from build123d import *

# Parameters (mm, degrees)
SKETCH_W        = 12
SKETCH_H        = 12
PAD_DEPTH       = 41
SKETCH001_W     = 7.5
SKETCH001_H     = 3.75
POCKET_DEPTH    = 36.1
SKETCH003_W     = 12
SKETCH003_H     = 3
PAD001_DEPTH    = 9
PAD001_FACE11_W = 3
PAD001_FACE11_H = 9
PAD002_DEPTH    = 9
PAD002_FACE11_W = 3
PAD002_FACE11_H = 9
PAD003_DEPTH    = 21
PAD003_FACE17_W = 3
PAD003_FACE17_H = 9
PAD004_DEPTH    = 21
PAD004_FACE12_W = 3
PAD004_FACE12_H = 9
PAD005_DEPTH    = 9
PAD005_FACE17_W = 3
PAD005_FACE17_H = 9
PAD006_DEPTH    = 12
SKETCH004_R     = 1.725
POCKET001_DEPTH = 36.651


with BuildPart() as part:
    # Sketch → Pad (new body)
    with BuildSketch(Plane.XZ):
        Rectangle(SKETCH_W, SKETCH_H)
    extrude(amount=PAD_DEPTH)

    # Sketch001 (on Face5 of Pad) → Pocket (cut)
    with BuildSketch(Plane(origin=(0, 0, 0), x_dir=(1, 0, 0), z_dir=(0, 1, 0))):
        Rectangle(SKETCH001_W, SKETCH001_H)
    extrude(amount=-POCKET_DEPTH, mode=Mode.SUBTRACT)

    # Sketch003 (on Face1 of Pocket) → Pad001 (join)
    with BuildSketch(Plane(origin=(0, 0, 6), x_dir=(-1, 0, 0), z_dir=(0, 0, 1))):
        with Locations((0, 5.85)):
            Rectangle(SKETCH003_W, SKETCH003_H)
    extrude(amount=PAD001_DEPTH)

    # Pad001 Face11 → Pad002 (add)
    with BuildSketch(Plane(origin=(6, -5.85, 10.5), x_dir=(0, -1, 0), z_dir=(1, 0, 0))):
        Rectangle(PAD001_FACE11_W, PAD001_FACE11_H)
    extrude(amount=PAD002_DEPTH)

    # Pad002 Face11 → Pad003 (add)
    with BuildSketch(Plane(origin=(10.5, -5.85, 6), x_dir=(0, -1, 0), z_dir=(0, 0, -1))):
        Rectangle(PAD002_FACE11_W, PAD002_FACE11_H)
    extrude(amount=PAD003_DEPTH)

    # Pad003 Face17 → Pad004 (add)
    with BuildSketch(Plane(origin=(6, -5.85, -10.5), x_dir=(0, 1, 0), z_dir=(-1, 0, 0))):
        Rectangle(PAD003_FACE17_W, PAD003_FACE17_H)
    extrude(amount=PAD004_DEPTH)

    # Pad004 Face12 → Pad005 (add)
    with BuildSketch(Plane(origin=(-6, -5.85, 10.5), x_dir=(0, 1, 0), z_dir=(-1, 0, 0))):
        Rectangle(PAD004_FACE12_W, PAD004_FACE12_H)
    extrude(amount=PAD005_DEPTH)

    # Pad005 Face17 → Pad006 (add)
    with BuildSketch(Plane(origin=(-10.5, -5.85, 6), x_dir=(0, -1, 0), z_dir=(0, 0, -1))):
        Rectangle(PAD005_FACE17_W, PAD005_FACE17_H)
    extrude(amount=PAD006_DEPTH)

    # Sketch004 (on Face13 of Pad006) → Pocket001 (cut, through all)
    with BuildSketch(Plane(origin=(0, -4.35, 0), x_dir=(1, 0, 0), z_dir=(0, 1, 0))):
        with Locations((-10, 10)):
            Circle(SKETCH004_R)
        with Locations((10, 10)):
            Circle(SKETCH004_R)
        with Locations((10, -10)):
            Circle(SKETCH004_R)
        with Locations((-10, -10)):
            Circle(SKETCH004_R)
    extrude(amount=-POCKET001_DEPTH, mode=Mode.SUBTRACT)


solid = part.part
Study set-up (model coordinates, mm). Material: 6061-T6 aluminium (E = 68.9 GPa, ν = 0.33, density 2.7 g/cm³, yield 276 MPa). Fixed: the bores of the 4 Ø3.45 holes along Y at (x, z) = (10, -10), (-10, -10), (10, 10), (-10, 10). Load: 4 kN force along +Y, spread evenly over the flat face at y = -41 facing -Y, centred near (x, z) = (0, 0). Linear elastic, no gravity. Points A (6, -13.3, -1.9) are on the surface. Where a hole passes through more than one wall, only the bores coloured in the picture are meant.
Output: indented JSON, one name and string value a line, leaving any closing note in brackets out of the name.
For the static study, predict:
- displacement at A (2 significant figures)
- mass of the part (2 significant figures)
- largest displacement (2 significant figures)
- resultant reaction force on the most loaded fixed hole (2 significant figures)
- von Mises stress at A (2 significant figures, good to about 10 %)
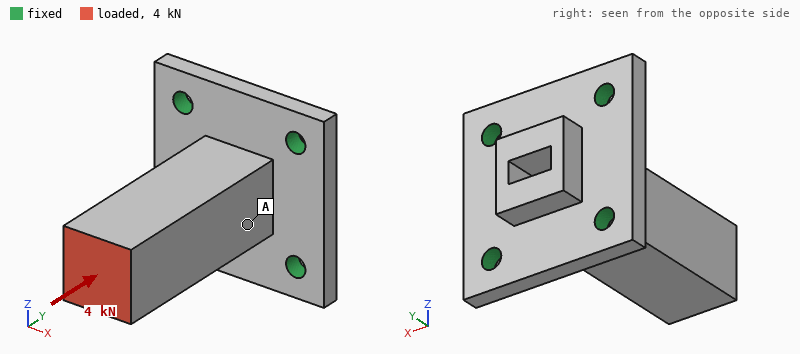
{
  "displacement at A": "30 µm",
  "mass of the part": "19 g",
  "largest displacement": "44 µm",
  "resultant reaction force on the most loaded fixed hole": "1.0 kN",
  "von Mises stress at A": "29 MPa"
}
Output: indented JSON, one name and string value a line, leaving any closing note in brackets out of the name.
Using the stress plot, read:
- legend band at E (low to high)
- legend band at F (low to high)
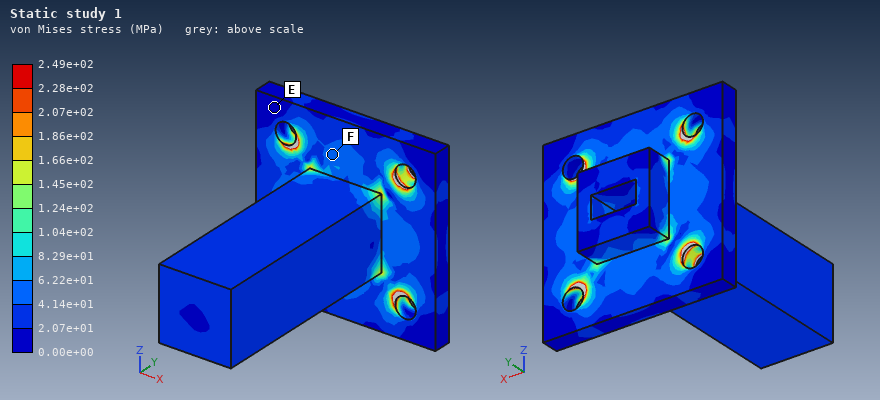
{
  "legend band at E": "0.00e+00 to 2.07e+01 MPa",
  "legend band at F": "4.14e+01 to 6.22e+01 MPa"
}
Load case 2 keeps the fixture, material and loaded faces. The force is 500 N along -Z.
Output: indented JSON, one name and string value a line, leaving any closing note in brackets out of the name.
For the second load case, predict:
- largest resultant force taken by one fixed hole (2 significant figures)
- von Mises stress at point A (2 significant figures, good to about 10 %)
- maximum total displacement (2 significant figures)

{
  "largest resultant force taken by one fixed hole": "550 N",
  "von Mises stress at point A": "19 MPa",
  "maximum total displacement": "0.14 mm"
}
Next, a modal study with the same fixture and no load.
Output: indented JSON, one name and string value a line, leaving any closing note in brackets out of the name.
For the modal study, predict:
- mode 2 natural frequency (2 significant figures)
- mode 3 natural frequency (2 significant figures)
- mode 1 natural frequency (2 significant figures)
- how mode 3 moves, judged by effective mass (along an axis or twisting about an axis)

{
  "mode 2 natural frequency": "5100 Hz",
  "mode 3 natural frequency": "15 kHz",
  "mode 1 natural frequency": "5000 Hz",
  "how mode 3 moves, judged by effective mass": "along Y"
}
